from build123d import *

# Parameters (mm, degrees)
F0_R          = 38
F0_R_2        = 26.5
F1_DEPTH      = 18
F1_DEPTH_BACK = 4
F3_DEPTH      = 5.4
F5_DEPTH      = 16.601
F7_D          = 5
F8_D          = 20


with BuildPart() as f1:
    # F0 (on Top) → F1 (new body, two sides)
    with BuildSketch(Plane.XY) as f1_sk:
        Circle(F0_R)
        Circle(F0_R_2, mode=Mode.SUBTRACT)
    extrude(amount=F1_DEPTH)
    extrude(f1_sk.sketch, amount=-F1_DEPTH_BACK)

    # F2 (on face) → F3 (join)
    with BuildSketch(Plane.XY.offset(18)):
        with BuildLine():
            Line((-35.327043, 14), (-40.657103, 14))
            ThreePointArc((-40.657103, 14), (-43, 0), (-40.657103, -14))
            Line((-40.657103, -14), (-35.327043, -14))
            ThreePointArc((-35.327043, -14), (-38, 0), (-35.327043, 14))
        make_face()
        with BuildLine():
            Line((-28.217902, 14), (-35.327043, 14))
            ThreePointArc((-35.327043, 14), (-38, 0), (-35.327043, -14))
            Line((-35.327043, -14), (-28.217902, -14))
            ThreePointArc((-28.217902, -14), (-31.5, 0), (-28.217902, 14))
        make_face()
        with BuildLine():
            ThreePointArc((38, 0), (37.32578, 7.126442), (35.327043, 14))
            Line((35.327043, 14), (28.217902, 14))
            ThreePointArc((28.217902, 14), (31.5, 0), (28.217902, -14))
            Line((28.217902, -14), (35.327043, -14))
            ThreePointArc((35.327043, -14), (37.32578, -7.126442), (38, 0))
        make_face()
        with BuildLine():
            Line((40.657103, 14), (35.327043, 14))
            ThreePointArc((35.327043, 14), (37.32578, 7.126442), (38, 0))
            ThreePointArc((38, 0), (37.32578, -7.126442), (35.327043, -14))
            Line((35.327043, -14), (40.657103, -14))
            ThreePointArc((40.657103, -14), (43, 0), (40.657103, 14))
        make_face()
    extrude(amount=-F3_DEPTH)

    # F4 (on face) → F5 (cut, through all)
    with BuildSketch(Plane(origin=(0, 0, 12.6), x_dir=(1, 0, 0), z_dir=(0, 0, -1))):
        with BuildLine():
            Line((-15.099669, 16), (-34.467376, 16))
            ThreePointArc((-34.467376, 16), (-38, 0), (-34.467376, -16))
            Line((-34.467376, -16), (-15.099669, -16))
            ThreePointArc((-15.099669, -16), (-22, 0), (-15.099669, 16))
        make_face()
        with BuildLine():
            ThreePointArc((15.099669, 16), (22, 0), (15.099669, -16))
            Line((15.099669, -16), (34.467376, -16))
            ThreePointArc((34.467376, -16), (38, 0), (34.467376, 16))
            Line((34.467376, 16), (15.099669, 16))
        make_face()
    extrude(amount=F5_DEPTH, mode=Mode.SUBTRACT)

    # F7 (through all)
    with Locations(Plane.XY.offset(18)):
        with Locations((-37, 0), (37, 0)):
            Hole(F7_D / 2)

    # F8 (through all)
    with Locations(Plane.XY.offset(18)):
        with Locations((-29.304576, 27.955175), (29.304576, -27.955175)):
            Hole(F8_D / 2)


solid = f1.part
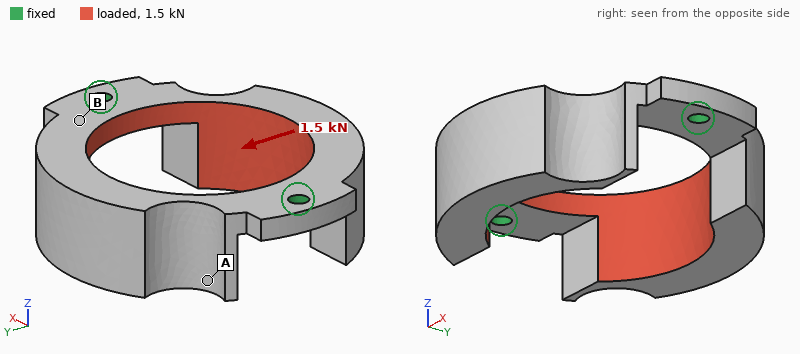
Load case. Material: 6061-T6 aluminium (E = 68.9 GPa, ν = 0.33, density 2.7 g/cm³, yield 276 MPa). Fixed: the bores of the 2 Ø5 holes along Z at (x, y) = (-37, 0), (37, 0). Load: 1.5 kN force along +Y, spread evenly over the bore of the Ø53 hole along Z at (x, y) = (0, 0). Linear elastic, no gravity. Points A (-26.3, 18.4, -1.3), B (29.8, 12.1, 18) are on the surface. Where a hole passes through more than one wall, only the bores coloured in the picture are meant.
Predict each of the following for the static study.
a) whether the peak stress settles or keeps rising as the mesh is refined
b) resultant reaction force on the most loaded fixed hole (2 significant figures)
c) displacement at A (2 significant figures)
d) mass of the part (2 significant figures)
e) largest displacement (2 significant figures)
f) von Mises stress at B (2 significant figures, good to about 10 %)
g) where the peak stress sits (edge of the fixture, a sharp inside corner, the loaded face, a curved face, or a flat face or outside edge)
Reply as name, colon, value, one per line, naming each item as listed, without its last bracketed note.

whether the peak stress settles or keeps rising as the mesh is refined: keeps rising
resultant reaction force on the most loaded fixed hole: 750 N
displacement at A: 0.095 mm
mass of the part: 96 g
largest displacement: 0.18 mm
von Mises stress at B: 48 MPa
where the peak stress sits: edge of the fixture
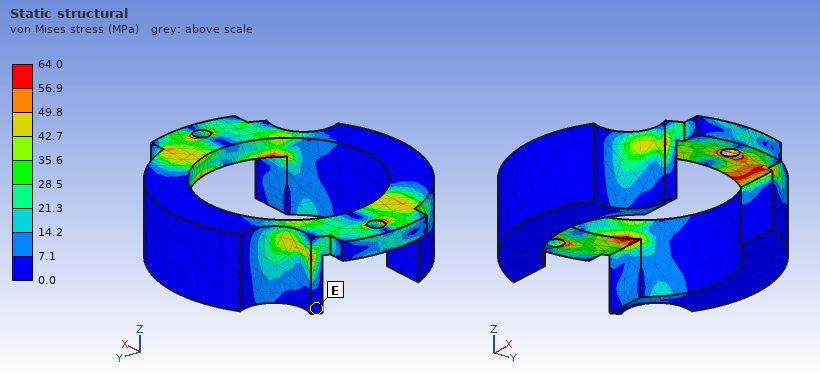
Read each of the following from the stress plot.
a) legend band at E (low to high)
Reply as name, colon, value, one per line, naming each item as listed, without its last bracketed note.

legend band at E: 0.0 to 7.1 MPa
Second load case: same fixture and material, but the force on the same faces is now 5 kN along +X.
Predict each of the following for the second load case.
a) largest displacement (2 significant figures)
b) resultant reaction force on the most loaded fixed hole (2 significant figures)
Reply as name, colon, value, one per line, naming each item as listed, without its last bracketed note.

largest displacement: 58 µm
resultant reaction force on the most loaded fixed hole: 2.5 kN
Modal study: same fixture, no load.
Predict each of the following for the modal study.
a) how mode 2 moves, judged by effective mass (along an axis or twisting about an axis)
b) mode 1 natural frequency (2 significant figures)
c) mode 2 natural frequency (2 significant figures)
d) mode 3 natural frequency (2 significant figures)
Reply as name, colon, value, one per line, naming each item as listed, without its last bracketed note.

how mode 2 moves, judged by effective mass: along Z
mode 1 natural frequency: 1200 Hz
mode 2 natural frequency: 1200 Hz
mode 3 natural frequency: 5000 Hz
